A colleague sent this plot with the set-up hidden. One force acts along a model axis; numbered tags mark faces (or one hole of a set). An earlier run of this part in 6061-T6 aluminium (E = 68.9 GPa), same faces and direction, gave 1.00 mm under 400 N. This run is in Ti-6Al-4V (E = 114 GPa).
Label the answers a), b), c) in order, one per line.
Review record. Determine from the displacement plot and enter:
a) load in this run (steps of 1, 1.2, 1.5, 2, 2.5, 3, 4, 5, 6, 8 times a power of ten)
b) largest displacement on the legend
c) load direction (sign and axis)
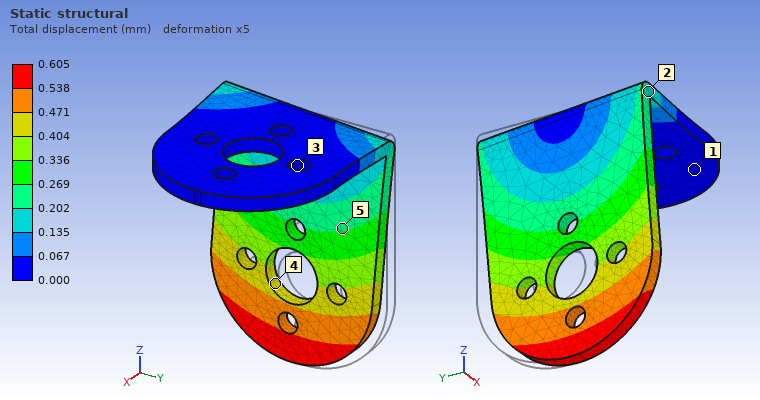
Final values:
a) 400 N
b) 0.605 mm
c) -Y
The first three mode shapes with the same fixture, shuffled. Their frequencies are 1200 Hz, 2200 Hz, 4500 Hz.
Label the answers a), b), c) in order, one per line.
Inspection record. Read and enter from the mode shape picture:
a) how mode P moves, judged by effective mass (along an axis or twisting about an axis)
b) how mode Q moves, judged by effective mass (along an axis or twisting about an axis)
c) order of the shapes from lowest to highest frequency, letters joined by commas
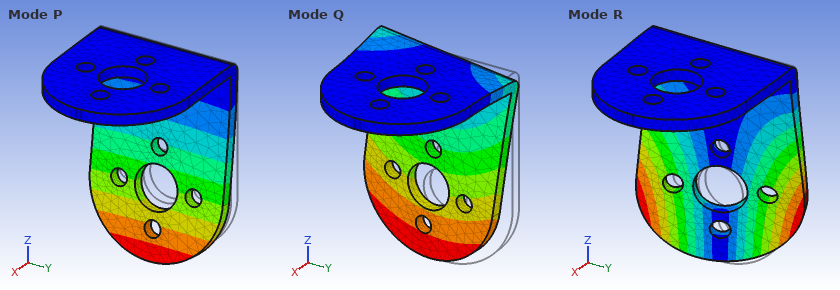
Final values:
a) along X
b) along Y
c) P, Q, R
